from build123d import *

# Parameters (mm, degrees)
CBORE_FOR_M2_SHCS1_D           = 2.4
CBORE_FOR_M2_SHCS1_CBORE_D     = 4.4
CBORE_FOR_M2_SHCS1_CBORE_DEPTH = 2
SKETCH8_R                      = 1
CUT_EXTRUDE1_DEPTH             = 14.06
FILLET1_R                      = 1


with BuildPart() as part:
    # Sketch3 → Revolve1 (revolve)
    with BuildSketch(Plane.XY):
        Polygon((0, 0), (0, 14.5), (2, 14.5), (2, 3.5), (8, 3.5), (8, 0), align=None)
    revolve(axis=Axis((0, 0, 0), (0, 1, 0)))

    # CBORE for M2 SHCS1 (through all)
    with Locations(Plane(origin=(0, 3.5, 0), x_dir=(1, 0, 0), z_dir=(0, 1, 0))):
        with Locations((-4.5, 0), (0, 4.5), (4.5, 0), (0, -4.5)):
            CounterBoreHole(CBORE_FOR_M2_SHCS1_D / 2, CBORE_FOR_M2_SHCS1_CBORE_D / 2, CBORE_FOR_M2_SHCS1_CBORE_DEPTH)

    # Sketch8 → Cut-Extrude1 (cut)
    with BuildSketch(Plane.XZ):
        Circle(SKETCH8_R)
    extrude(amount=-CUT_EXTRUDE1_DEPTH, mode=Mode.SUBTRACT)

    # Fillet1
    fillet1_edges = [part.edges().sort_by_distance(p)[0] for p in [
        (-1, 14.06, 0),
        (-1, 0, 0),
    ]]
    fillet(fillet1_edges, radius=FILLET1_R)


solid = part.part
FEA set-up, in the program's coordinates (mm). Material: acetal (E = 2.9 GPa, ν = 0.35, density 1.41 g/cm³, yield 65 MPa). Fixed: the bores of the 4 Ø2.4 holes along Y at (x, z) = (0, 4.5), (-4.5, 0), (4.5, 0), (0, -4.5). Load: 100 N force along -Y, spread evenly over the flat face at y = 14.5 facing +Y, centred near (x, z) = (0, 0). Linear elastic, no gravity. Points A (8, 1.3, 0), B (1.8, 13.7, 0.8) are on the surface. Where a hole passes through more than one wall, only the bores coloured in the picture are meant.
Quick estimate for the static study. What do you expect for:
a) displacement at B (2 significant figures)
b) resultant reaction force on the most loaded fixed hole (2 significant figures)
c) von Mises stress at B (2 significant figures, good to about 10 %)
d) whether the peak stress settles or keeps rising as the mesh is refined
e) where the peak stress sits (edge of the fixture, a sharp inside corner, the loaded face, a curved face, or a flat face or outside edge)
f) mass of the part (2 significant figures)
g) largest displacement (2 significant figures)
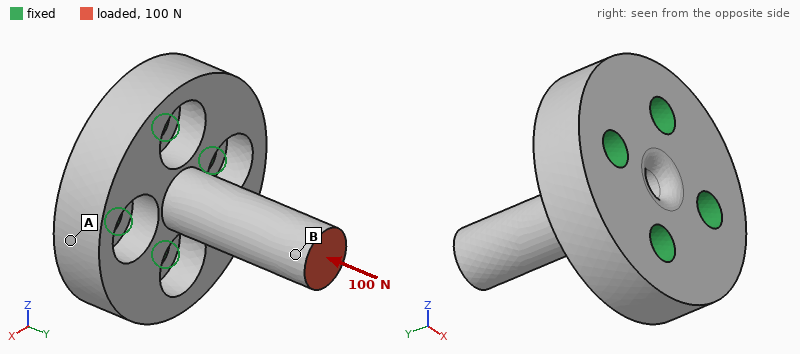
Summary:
48 µm
28 N
7.7 MPa
keeps rising
edge of the fixture
0.91 g
57 µm
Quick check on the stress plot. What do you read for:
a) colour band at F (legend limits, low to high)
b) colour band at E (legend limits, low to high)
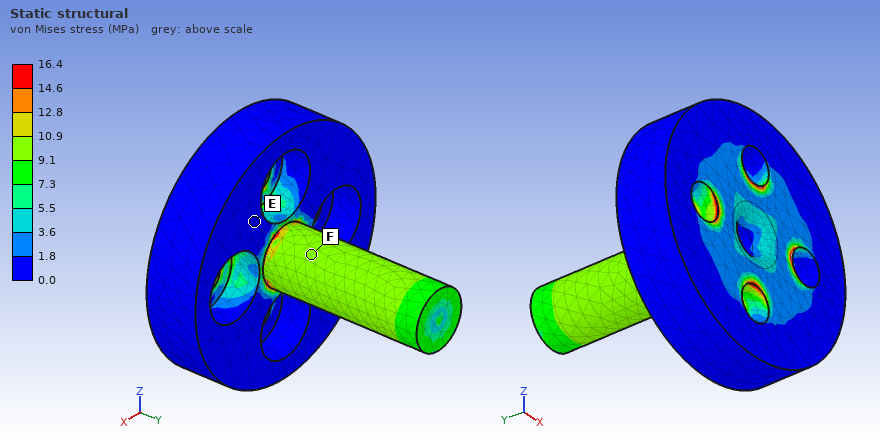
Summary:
9.1 to 10.9 MPa
0.0 to 1.8 MPa
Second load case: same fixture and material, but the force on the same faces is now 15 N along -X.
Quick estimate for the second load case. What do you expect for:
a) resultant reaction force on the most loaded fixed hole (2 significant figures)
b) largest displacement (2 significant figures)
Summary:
24 N
0.31 mm
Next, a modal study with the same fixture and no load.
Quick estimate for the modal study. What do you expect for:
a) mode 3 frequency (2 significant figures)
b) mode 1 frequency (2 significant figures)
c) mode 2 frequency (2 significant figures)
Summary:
18 kHz
5300 Hz
5300 Hz
